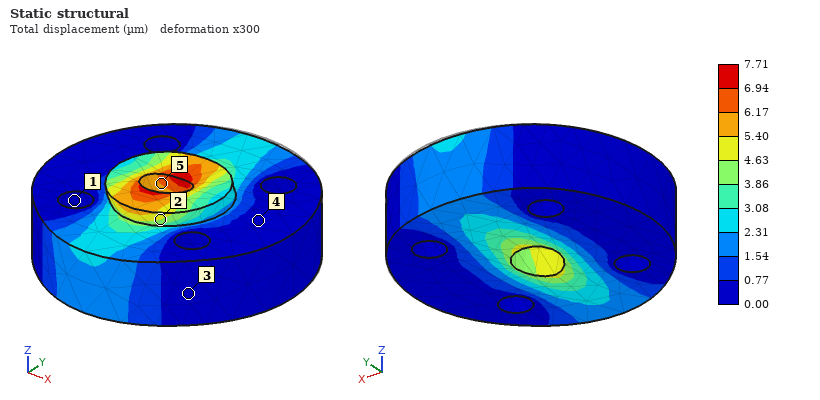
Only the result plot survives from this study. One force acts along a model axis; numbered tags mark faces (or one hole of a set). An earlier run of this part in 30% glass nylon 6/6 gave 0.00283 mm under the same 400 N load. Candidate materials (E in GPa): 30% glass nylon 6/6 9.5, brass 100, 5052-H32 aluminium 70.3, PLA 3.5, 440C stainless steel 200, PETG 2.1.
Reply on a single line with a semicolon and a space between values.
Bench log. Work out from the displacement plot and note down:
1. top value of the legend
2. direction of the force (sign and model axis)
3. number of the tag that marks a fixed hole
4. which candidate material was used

7.71 µm; -Y; 1; PLA
